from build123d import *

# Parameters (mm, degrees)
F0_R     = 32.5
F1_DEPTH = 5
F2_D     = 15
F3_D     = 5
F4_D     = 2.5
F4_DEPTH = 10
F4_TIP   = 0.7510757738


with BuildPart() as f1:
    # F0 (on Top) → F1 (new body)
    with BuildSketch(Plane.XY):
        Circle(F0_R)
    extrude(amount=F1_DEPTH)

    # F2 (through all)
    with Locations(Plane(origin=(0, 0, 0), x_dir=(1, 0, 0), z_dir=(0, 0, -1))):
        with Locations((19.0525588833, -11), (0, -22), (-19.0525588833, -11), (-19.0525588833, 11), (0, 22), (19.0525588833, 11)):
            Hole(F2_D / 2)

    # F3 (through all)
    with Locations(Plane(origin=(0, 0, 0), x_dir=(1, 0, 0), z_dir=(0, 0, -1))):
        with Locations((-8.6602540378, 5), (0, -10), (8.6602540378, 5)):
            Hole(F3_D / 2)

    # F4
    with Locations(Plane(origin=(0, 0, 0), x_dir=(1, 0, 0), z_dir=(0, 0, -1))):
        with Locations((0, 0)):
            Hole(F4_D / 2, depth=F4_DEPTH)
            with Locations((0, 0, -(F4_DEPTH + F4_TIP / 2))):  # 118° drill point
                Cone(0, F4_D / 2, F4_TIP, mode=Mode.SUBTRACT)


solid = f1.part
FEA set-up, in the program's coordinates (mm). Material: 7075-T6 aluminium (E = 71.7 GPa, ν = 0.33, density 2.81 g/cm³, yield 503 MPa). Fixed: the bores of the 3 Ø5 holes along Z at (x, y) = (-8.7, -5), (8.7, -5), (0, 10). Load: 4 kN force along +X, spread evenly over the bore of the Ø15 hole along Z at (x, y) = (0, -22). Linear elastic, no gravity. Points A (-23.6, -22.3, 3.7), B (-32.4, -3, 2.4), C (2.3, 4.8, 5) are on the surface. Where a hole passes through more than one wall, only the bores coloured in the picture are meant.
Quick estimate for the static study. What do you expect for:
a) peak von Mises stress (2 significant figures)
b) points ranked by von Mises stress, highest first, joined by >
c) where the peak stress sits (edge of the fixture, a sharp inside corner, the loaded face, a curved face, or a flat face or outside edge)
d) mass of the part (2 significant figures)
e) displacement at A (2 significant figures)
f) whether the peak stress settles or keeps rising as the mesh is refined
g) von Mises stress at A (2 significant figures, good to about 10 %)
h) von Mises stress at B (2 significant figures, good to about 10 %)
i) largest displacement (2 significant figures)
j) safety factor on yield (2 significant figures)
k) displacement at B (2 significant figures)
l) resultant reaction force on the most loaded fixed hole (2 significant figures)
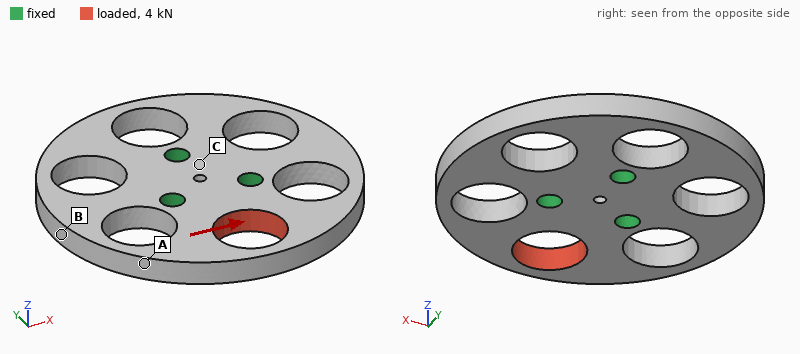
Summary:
150 MPa
A > B > C
the loaded face
31 g
52 µm
settles
70 MPa
29 MPa
67 µm
3.3
38 µm
3.4 kN
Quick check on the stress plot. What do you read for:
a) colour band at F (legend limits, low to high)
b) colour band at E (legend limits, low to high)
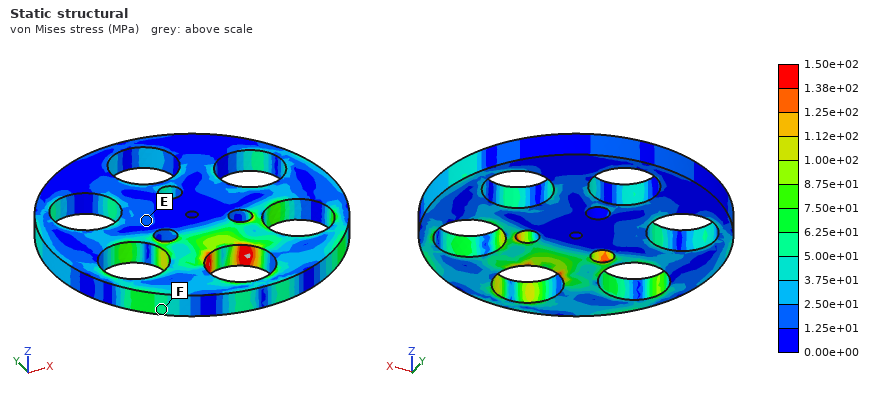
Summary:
5.00e+01 to 6.25e+01 MPa
1.25e+01 to 2.50e+01 MPa
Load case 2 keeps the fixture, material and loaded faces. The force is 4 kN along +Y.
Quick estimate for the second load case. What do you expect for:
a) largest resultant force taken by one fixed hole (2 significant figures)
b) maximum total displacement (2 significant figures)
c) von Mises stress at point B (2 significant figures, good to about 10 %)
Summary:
1.9 kN
31 µm
8.2 MPa
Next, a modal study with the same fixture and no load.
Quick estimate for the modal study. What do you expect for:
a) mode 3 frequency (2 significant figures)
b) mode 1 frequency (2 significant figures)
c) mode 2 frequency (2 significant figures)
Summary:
5500 Hz
5400 Hz
5400 Hz
